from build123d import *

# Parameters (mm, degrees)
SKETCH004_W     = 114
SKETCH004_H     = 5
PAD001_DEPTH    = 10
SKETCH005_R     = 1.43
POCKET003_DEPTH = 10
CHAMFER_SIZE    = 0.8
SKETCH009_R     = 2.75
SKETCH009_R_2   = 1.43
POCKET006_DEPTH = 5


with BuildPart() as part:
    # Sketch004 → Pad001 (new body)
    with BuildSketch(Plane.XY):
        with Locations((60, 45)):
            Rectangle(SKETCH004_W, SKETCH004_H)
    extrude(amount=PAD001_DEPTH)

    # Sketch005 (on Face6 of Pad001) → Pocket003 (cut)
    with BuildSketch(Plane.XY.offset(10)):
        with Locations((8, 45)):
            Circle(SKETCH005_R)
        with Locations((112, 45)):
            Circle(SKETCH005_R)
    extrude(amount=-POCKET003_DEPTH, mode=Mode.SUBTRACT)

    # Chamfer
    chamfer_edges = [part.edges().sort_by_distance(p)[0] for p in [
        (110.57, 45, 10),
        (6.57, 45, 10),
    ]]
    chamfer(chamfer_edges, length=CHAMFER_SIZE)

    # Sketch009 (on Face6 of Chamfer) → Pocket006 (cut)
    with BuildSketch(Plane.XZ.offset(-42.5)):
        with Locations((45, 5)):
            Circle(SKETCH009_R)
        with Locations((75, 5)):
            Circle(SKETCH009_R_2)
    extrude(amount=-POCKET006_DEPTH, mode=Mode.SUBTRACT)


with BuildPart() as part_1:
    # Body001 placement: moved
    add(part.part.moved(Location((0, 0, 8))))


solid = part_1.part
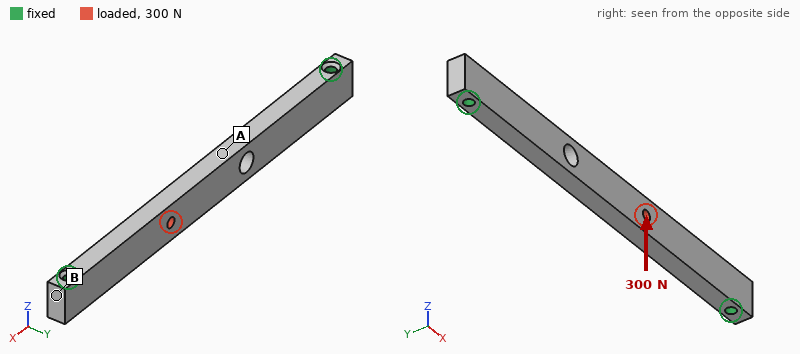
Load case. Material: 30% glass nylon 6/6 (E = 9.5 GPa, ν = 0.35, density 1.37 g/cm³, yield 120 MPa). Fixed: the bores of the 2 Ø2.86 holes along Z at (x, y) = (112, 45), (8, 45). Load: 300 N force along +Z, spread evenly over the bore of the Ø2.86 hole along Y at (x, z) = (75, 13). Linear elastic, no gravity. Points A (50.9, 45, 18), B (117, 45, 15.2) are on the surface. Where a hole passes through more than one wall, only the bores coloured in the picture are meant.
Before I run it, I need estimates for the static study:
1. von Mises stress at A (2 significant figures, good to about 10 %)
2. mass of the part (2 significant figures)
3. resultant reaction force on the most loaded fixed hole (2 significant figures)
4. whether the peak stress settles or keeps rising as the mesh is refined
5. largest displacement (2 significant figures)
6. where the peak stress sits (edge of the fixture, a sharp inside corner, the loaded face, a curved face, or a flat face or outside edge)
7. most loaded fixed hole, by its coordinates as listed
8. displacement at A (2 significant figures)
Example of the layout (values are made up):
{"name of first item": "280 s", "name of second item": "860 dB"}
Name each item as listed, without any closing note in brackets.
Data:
{"von Mises stress at A": "16 MPa", "mass of the part": "7.4 g", "resultant reaction force on the most loaded fixed hole": "210 N", "whether the peak stress settles or keeps rising as the mesh is refined": "keeps rising", "largest displacement": "0.41 mm", "where the peak stress sits": "edge of the fixture", "most loaded fixed hole, by its coordinates as listed": "(112, 45)", "displacement at A": "0.33 mm"}
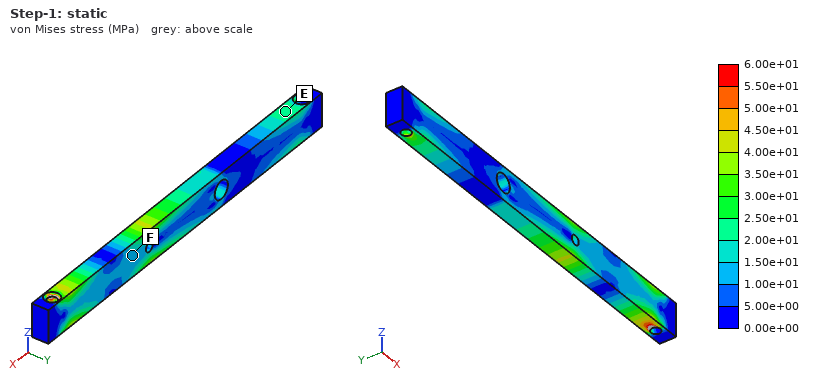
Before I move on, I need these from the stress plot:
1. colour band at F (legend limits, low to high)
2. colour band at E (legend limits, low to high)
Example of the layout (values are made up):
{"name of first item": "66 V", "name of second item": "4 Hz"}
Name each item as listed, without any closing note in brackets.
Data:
{"colour band at F": "1.00e+01 to 1.50e+01 MPa", "colour band at E": "2.00e+01 to 2.50e+01 MPa"}
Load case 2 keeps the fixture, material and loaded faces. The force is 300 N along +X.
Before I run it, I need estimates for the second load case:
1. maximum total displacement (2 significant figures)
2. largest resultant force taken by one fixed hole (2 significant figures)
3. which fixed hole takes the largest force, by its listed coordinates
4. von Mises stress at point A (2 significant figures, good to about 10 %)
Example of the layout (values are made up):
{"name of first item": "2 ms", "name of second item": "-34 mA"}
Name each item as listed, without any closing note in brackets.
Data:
{"maximum total displacement": "17 µm", "largest resultant force taken by one fixed hole": "200 N", "which fixed hole takes the largest force, by its listed coordinates": "(112, 45)", "von Mises stress at point A": "3.3 MPa"}
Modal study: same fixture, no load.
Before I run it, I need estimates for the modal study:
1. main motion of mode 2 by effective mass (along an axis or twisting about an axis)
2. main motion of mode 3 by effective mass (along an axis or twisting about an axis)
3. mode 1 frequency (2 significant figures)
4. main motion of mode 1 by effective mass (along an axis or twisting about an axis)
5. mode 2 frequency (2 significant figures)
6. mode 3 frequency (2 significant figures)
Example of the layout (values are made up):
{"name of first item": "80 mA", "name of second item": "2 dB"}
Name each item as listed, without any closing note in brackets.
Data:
{"main motion of mode 2 by effective mass": "along Z", "main motion of mode 3 by effective mass": "twisting about Z", "mode 1 frequency": "1200 Hz", "main motion of mode 1 by effective mass": "along Y", "mode 2 frequency": "2400 Hz", "mode 3 frequency": "3300 Hz"}
